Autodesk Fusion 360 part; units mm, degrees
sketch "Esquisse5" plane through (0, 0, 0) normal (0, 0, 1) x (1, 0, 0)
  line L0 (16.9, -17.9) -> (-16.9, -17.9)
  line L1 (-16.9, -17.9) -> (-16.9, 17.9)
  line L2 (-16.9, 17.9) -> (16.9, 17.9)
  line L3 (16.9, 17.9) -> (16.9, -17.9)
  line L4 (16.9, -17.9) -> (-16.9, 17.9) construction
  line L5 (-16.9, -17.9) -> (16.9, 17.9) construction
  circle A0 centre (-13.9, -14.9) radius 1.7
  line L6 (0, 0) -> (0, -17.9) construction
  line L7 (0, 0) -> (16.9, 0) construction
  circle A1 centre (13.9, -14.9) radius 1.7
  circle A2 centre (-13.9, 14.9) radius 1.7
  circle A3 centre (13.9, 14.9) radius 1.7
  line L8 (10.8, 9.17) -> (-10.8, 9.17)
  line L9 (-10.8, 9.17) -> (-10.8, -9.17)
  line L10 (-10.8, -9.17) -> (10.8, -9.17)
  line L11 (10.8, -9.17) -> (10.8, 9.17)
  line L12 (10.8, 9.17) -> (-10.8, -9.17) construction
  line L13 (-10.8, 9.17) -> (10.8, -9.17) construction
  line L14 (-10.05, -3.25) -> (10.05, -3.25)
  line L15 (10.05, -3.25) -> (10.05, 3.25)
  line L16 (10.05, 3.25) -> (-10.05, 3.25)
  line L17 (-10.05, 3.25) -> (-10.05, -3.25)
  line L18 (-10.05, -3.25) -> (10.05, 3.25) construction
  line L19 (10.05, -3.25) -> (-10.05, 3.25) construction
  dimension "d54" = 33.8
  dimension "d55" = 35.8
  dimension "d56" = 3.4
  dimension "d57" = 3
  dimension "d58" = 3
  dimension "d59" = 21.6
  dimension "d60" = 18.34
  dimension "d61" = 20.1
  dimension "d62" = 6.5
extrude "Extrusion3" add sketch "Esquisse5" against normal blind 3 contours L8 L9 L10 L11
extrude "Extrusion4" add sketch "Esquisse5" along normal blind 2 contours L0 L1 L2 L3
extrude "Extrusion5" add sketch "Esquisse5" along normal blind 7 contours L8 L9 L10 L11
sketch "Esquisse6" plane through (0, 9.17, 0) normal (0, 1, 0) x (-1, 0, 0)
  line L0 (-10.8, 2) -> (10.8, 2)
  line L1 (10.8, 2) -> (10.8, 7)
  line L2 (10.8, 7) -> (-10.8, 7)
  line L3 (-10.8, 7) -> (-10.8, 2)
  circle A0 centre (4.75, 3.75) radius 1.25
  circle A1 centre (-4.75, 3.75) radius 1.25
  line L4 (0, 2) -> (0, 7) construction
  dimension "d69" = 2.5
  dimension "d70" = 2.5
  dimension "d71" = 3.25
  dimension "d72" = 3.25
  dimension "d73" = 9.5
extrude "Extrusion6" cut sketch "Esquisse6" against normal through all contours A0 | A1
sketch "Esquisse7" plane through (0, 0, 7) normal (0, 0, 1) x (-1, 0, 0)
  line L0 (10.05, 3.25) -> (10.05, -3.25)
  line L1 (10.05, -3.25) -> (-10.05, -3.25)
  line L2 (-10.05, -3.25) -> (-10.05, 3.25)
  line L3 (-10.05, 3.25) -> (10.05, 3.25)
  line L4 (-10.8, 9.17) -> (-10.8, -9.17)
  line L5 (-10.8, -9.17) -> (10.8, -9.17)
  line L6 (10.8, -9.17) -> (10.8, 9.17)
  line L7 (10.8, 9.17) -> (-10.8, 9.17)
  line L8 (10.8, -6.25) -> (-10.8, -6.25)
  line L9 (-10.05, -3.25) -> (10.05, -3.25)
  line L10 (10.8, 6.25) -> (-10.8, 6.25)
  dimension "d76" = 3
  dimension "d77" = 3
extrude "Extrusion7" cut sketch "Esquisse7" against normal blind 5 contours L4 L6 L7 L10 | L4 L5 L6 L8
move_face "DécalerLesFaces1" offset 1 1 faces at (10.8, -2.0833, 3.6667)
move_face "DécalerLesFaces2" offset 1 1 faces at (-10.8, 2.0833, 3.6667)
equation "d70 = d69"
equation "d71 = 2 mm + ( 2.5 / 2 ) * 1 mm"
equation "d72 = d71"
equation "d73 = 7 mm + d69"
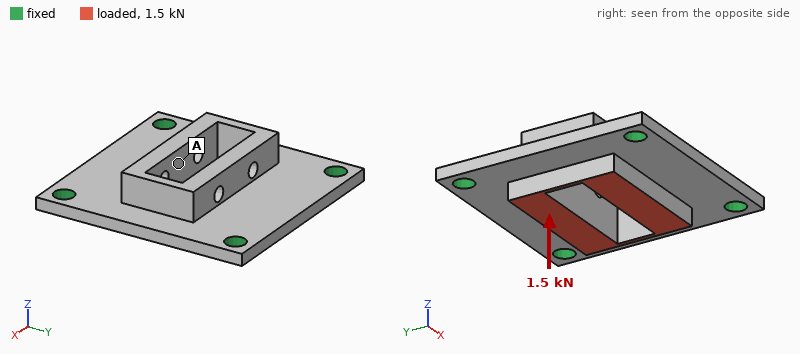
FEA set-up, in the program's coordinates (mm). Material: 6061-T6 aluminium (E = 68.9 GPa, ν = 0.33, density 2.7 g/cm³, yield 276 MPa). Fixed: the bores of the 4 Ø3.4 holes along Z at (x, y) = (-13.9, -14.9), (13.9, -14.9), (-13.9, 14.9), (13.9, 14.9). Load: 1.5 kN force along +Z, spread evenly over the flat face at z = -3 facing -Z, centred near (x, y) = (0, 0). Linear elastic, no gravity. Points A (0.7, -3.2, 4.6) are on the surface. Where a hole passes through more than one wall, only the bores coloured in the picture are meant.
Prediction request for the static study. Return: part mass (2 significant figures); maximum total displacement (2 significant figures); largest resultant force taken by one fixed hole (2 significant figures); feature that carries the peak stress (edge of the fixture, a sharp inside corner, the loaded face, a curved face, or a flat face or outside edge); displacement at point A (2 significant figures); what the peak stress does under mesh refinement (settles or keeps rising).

9.8 g
59 µm
380 N
edge of the fixture
58 µm
keeps rising
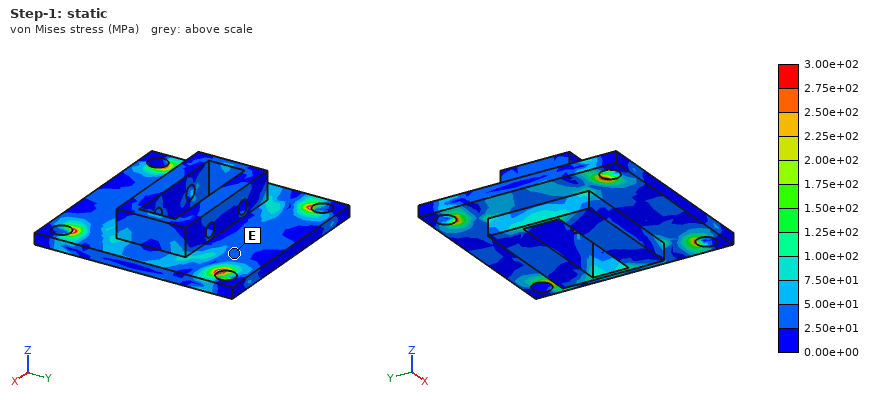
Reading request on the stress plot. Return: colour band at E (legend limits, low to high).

2.50e+01 to 5.00e+01 MPa
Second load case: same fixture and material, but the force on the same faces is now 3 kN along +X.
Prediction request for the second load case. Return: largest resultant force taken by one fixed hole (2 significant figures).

860 N
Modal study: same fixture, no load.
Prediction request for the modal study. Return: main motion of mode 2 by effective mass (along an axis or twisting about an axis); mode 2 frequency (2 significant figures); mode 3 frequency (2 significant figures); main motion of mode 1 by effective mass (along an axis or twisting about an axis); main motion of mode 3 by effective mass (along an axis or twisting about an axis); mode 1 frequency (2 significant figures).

twisting about Y
15 kHz
17 kHz
along Z
twisting about X
10 kHz
